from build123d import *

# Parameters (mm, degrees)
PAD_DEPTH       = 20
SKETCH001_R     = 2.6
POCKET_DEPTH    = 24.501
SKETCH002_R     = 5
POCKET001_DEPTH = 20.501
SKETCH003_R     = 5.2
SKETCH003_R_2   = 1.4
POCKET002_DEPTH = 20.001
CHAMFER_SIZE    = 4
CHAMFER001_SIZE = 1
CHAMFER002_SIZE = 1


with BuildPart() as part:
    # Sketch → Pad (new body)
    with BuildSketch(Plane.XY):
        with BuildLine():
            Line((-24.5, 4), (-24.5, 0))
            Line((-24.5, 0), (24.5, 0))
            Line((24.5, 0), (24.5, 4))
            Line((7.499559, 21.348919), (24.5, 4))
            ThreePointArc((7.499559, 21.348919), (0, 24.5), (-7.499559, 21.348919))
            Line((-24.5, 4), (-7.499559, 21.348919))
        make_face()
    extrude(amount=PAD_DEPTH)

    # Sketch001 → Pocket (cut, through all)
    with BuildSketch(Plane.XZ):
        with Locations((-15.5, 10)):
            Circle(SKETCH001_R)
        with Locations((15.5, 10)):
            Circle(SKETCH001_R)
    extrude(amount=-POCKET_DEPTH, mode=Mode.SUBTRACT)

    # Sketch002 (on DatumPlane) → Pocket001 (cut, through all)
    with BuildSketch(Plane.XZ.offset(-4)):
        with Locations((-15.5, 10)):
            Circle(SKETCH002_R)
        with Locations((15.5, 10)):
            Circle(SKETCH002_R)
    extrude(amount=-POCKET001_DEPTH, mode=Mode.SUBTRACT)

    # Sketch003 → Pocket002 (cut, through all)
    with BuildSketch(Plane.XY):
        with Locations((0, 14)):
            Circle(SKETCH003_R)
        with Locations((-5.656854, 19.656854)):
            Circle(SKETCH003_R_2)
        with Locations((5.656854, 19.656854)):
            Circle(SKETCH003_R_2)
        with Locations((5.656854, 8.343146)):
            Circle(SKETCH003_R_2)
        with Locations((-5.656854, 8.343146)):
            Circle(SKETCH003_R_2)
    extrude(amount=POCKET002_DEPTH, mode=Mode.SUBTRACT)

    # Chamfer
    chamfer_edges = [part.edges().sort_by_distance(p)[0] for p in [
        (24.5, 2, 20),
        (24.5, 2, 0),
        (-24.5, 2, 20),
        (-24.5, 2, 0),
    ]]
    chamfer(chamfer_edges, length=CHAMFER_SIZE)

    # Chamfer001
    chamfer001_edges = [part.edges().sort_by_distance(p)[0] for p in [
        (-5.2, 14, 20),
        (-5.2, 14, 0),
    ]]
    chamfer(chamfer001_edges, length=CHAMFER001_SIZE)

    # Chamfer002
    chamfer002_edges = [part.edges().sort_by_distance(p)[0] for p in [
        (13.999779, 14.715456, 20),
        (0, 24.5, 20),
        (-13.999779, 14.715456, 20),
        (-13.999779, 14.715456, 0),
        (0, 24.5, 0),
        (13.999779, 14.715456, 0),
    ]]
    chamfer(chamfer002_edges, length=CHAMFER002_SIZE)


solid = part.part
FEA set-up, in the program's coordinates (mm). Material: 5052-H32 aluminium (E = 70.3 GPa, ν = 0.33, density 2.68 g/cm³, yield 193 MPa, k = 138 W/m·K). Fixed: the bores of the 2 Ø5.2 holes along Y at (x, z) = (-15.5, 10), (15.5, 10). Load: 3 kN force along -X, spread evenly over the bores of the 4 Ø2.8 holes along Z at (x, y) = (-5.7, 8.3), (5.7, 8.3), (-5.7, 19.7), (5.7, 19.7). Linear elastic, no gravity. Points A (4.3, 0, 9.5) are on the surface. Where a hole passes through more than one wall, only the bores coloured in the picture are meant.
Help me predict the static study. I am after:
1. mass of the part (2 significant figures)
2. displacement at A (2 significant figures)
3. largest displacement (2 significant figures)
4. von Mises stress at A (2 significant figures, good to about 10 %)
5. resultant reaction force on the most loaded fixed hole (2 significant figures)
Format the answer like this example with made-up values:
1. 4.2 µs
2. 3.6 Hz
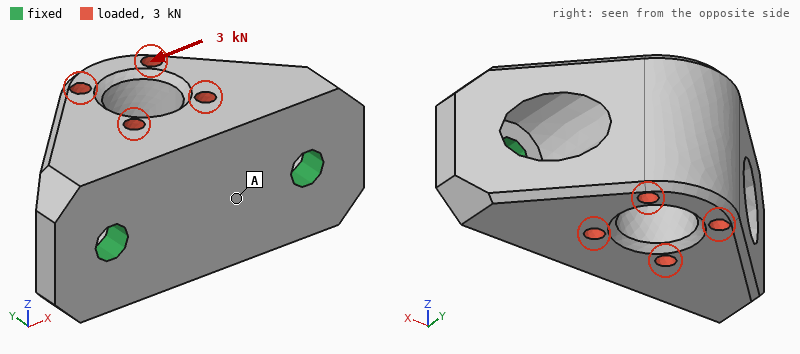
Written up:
1. 31 g
2. 1.9 µm
3. 11 µm
4. 7.7 MPa
5. 1.9 kN
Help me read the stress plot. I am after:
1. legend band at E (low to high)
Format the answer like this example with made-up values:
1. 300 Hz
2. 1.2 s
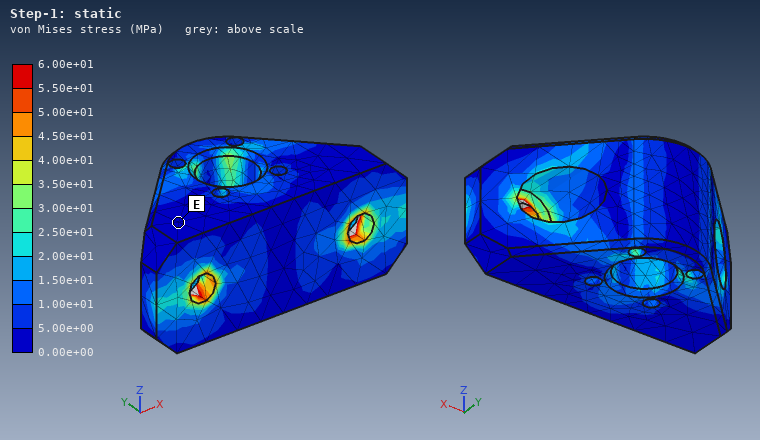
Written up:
1. 0.00e+00 to 5.00e+00 MPa
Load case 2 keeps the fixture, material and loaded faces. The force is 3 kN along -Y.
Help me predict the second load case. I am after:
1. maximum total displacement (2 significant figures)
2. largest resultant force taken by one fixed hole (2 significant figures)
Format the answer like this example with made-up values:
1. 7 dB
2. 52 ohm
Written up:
1. 7.6 µm
2. 1.6 kN
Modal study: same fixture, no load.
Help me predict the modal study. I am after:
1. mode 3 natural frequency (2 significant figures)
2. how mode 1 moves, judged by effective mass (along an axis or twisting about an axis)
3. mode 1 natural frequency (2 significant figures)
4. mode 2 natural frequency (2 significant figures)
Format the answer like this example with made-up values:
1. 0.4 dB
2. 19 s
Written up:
1. 22 kHz
2. along Z
3. 8200 Hz
4. 22 kHz
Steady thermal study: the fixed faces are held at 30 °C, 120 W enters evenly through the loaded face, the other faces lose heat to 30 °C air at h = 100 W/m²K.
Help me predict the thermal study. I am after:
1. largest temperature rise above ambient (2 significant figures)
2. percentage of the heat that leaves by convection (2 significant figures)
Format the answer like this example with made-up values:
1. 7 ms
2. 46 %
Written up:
1. 50 K
2. 10 %
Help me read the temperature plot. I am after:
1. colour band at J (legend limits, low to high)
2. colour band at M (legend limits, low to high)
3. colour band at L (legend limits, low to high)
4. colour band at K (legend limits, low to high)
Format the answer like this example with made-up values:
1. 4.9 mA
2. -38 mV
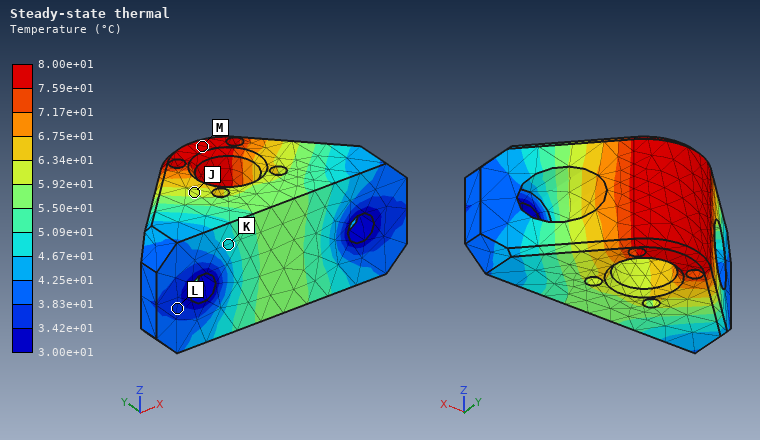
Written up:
1. 5.92e+01 to 6.34e+01 °C
2. 7.59e+01 to 8.00e+01 °C
3. 3.42e+01 to 3.83e+01 °C
4. 4.67e+01 to 5.09e+01 °C
